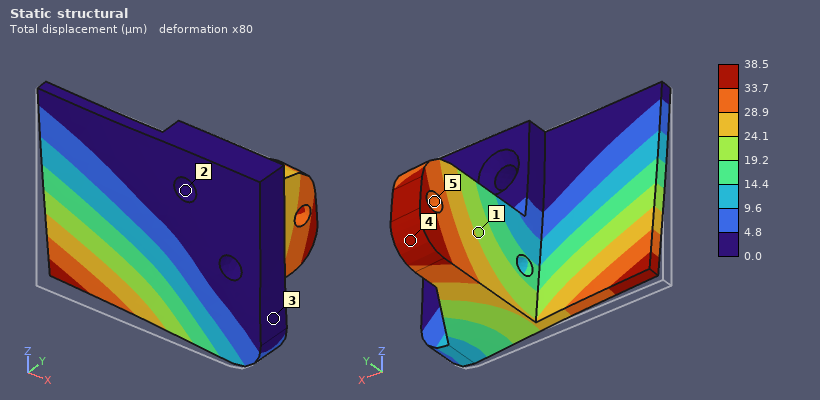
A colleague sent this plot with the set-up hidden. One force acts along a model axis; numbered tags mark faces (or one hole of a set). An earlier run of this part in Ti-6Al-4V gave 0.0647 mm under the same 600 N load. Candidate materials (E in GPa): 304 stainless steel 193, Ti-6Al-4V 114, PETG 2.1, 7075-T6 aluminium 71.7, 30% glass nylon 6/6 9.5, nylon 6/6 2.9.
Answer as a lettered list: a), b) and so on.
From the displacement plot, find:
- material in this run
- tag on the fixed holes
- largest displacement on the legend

a) 304 stainless steel
b) 2
c) 38.5 µm
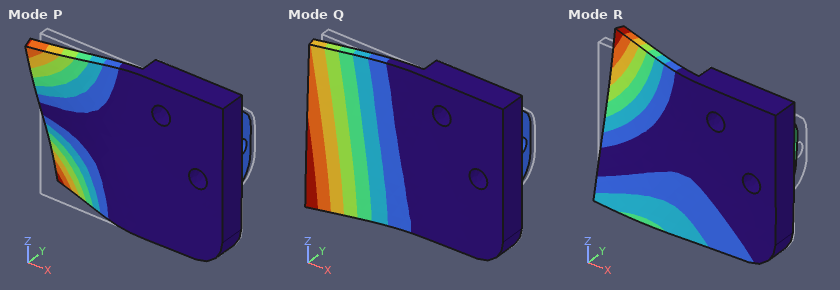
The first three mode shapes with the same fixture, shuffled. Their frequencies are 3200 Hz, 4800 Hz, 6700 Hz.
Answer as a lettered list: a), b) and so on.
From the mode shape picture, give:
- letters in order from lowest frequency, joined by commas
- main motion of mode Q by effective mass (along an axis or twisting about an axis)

a) Q, R, P
b) along Y
